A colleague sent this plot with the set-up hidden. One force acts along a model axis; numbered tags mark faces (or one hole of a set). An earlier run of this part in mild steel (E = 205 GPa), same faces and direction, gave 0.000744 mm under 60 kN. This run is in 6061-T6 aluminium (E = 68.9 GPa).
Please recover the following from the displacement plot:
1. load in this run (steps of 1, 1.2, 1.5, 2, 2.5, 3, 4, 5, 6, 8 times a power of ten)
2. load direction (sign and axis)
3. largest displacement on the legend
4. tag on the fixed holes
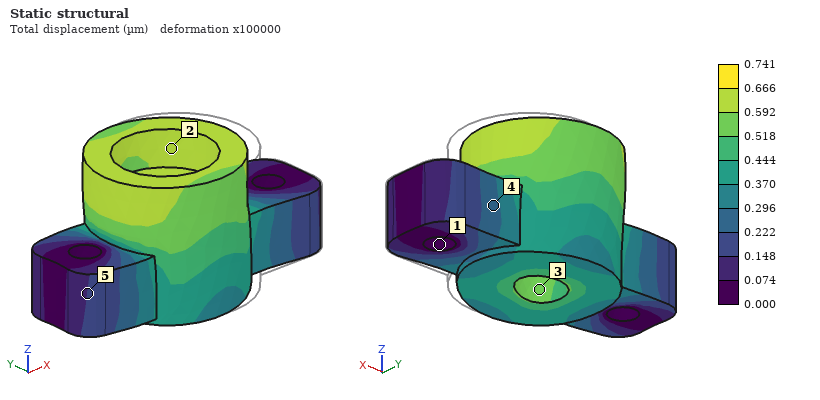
20 kN
-X
0.741 µm
1
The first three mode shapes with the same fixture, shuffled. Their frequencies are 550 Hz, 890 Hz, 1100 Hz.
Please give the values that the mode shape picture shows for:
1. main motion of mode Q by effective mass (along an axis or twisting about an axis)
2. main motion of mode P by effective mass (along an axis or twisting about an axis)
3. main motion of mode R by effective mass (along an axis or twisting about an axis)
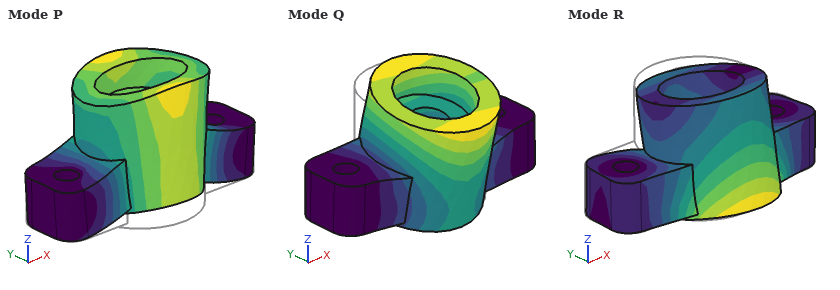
along Y
along Z
along Y
